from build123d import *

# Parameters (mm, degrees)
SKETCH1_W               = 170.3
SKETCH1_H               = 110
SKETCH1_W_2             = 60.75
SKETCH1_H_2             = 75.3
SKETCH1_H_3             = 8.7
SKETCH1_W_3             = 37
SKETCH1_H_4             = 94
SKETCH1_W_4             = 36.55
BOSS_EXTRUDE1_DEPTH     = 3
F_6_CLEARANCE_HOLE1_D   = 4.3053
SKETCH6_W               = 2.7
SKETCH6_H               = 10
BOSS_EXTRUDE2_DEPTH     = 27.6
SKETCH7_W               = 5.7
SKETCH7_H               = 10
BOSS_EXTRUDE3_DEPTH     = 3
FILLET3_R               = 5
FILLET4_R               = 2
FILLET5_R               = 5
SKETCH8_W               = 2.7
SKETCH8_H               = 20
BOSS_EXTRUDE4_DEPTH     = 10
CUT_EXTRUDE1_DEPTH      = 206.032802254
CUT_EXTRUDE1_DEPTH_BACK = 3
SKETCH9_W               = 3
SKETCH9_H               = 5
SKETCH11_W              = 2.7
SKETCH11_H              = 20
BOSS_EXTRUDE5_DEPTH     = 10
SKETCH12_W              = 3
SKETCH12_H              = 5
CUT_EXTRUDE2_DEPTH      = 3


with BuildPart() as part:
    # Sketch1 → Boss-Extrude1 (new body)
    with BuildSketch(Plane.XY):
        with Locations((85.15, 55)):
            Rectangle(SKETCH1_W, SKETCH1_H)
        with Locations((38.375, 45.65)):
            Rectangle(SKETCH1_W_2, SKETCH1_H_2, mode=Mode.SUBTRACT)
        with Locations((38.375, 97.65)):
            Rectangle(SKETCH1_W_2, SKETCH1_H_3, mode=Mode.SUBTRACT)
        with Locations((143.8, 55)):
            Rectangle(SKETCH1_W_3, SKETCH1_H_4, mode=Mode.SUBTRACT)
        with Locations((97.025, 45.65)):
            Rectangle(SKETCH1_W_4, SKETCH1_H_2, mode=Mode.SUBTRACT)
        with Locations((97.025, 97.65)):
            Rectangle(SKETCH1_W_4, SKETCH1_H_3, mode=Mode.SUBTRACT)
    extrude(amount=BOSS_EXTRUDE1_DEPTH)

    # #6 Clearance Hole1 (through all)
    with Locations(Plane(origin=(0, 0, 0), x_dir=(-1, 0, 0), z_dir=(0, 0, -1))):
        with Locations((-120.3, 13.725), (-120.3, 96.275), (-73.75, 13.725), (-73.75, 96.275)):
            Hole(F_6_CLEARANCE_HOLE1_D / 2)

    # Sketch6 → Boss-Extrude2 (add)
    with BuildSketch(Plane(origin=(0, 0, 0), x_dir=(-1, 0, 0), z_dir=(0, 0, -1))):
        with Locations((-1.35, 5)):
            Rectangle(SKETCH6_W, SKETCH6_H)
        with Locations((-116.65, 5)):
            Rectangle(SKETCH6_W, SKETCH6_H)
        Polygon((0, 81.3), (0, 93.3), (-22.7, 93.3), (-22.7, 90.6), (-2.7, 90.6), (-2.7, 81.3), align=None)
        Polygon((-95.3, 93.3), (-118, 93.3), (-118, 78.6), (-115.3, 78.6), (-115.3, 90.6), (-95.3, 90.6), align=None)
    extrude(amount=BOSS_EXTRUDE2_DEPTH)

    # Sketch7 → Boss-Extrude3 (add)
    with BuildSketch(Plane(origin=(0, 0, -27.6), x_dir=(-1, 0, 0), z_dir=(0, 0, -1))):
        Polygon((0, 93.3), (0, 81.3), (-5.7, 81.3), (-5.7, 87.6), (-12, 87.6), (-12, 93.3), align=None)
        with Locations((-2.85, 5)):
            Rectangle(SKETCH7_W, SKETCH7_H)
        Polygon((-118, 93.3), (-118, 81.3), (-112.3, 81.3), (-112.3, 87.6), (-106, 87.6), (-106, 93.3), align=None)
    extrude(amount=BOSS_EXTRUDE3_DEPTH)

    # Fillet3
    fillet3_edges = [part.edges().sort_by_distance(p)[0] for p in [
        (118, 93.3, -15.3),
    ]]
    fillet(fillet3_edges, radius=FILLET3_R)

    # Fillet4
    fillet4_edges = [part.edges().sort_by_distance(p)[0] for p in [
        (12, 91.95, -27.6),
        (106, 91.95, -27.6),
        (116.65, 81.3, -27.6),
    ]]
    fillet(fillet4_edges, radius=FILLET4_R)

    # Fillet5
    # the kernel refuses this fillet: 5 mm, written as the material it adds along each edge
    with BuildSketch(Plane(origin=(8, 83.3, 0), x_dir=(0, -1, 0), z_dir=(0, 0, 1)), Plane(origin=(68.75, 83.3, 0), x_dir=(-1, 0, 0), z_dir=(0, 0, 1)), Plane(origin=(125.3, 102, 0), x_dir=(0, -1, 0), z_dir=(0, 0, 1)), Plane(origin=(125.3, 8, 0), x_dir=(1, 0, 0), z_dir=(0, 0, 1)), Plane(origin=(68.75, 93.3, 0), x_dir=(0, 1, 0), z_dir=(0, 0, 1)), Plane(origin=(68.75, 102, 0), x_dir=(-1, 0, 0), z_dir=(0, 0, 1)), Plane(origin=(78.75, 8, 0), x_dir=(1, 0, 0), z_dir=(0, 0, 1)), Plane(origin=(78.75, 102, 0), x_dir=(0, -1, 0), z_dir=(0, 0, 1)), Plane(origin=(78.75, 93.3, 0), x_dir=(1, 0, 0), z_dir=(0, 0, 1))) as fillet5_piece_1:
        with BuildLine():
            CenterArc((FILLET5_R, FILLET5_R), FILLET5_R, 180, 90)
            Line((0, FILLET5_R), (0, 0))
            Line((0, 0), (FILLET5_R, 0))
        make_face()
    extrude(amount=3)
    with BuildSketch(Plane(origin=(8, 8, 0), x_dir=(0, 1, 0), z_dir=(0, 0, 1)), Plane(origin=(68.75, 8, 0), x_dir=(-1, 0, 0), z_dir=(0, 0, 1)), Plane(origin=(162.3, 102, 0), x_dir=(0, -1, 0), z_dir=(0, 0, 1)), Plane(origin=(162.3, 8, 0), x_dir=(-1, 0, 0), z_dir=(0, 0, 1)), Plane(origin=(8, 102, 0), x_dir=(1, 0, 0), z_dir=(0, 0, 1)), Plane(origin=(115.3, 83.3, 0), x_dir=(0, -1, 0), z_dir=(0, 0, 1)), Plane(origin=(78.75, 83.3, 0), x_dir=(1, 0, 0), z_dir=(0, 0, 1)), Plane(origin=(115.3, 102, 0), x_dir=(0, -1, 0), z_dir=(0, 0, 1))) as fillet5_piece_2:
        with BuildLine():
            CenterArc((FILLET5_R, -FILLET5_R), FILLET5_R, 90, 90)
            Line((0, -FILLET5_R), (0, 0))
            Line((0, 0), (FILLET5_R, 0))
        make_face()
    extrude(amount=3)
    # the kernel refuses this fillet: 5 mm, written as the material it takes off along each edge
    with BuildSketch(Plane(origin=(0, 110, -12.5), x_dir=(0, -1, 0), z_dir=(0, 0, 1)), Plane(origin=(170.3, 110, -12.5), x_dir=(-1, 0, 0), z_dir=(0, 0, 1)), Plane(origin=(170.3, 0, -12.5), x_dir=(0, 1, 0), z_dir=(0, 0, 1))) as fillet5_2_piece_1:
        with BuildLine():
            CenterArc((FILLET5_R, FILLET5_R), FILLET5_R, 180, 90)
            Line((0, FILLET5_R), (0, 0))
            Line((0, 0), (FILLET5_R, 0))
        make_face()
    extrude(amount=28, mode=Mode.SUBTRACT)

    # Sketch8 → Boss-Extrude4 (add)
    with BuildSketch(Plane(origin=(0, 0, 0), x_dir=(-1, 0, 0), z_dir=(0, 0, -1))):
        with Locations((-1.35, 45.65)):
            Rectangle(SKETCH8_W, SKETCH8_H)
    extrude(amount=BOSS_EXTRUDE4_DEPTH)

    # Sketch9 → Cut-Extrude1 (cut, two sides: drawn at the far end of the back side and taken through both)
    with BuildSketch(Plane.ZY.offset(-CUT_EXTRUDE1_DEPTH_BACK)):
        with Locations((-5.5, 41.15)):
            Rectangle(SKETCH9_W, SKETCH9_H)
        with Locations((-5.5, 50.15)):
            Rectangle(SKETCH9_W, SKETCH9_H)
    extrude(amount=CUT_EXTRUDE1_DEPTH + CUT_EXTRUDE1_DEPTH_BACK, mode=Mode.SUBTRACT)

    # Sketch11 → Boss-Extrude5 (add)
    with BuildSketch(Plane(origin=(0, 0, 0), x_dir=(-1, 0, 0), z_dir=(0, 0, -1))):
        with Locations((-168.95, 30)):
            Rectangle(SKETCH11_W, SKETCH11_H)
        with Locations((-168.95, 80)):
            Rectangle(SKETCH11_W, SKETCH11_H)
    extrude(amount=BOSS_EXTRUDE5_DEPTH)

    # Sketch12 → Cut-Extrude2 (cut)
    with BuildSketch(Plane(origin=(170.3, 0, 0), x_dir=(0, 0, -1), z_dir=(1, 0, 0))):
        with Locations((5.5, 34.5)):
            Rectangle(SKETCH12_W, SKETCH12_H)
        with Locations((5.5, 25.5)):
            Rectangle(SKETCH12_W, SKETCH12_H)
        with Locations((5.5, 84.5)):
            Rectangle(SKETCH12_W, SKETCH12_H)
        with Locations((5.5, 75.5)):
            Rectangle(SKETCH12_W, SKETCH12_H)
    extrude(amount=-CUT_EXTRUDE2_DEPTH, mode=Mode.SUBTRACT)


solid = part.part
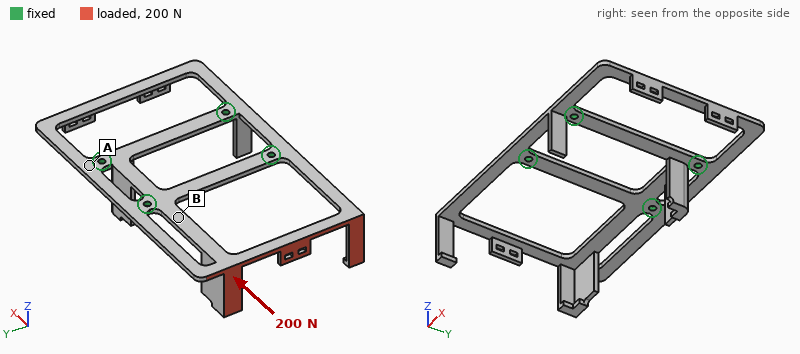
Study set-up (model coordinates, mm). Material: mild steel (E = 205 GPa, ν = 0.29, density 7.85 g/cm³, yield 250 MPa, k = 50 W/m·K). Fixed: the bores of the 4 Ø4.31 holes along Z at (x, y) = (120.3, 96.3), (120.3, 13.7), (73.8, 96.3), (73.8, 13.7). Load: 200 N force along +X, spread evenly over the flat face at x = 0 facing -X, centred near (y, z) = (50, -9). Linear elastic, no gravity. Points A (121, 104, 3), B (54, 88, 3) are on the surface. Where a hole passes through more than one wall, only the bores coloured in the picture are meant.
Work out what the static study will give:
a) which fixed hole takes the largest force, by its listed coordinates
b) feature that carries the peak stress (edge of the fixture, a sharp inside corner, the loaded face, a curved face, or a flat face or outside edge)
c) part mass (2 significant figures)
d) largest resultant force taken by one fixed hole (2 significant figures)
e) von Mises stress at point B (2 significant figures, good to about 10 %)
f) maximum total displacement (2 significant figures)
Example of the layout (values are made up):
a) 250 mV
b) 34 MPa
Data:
a) (73.8, 96.3)
b) a curved face
c) 230 g
d) 89 N
e) 50 MPa
f) 0.73 mm
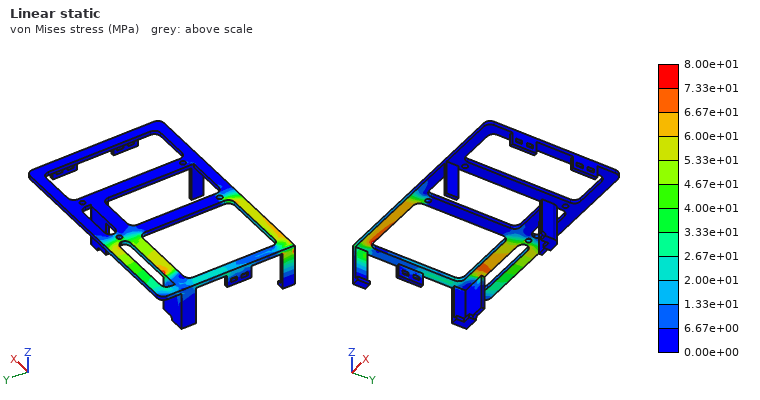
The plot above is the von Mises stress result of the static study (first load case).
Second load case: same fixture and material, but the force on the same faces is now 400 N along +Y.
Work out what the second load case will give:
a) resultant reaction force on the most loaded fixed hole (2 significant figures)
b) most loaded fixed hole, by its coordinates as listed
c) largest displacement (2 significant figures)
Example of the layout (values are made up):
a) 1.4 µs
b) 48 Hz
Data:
a) 460 N
b) (73.8, 96.3)
c) 0.76 mm
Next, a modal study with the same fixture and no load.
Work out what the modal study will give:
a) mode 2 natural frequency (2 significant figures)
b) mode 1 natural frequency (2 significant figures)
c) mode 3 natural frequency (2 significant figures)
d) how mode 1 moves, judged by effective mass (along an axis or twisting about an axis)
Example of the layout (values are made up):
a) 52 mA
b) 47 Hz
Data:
a) 380 Hz
b) 210 Hz
c) 400 Hz
d) along Z
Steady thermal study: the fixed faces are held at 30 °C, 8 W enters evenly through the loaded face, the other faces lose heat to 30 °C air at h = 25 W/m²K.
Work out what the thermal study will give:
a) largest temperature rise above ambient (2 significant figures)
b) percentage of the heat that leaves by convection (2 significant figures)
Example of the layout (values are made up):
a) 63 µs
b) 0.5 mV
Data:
a) 63 K
b) 83 %
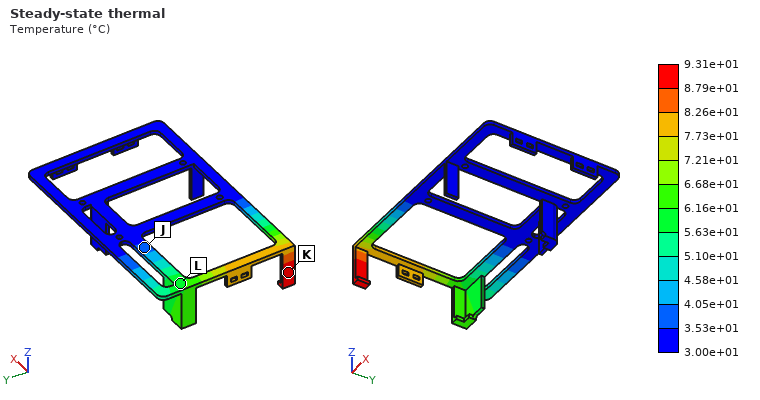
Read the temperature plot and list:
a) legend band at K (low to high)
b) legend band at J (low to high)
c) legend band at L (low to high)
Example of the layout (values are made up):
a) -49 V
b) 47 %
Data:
a) 8.79e+01 to 9.31e+01 °C
b) 3.53e+01 to 4.05e+01 °C
c) 5.63e+01 to 6.16e+01 °C
